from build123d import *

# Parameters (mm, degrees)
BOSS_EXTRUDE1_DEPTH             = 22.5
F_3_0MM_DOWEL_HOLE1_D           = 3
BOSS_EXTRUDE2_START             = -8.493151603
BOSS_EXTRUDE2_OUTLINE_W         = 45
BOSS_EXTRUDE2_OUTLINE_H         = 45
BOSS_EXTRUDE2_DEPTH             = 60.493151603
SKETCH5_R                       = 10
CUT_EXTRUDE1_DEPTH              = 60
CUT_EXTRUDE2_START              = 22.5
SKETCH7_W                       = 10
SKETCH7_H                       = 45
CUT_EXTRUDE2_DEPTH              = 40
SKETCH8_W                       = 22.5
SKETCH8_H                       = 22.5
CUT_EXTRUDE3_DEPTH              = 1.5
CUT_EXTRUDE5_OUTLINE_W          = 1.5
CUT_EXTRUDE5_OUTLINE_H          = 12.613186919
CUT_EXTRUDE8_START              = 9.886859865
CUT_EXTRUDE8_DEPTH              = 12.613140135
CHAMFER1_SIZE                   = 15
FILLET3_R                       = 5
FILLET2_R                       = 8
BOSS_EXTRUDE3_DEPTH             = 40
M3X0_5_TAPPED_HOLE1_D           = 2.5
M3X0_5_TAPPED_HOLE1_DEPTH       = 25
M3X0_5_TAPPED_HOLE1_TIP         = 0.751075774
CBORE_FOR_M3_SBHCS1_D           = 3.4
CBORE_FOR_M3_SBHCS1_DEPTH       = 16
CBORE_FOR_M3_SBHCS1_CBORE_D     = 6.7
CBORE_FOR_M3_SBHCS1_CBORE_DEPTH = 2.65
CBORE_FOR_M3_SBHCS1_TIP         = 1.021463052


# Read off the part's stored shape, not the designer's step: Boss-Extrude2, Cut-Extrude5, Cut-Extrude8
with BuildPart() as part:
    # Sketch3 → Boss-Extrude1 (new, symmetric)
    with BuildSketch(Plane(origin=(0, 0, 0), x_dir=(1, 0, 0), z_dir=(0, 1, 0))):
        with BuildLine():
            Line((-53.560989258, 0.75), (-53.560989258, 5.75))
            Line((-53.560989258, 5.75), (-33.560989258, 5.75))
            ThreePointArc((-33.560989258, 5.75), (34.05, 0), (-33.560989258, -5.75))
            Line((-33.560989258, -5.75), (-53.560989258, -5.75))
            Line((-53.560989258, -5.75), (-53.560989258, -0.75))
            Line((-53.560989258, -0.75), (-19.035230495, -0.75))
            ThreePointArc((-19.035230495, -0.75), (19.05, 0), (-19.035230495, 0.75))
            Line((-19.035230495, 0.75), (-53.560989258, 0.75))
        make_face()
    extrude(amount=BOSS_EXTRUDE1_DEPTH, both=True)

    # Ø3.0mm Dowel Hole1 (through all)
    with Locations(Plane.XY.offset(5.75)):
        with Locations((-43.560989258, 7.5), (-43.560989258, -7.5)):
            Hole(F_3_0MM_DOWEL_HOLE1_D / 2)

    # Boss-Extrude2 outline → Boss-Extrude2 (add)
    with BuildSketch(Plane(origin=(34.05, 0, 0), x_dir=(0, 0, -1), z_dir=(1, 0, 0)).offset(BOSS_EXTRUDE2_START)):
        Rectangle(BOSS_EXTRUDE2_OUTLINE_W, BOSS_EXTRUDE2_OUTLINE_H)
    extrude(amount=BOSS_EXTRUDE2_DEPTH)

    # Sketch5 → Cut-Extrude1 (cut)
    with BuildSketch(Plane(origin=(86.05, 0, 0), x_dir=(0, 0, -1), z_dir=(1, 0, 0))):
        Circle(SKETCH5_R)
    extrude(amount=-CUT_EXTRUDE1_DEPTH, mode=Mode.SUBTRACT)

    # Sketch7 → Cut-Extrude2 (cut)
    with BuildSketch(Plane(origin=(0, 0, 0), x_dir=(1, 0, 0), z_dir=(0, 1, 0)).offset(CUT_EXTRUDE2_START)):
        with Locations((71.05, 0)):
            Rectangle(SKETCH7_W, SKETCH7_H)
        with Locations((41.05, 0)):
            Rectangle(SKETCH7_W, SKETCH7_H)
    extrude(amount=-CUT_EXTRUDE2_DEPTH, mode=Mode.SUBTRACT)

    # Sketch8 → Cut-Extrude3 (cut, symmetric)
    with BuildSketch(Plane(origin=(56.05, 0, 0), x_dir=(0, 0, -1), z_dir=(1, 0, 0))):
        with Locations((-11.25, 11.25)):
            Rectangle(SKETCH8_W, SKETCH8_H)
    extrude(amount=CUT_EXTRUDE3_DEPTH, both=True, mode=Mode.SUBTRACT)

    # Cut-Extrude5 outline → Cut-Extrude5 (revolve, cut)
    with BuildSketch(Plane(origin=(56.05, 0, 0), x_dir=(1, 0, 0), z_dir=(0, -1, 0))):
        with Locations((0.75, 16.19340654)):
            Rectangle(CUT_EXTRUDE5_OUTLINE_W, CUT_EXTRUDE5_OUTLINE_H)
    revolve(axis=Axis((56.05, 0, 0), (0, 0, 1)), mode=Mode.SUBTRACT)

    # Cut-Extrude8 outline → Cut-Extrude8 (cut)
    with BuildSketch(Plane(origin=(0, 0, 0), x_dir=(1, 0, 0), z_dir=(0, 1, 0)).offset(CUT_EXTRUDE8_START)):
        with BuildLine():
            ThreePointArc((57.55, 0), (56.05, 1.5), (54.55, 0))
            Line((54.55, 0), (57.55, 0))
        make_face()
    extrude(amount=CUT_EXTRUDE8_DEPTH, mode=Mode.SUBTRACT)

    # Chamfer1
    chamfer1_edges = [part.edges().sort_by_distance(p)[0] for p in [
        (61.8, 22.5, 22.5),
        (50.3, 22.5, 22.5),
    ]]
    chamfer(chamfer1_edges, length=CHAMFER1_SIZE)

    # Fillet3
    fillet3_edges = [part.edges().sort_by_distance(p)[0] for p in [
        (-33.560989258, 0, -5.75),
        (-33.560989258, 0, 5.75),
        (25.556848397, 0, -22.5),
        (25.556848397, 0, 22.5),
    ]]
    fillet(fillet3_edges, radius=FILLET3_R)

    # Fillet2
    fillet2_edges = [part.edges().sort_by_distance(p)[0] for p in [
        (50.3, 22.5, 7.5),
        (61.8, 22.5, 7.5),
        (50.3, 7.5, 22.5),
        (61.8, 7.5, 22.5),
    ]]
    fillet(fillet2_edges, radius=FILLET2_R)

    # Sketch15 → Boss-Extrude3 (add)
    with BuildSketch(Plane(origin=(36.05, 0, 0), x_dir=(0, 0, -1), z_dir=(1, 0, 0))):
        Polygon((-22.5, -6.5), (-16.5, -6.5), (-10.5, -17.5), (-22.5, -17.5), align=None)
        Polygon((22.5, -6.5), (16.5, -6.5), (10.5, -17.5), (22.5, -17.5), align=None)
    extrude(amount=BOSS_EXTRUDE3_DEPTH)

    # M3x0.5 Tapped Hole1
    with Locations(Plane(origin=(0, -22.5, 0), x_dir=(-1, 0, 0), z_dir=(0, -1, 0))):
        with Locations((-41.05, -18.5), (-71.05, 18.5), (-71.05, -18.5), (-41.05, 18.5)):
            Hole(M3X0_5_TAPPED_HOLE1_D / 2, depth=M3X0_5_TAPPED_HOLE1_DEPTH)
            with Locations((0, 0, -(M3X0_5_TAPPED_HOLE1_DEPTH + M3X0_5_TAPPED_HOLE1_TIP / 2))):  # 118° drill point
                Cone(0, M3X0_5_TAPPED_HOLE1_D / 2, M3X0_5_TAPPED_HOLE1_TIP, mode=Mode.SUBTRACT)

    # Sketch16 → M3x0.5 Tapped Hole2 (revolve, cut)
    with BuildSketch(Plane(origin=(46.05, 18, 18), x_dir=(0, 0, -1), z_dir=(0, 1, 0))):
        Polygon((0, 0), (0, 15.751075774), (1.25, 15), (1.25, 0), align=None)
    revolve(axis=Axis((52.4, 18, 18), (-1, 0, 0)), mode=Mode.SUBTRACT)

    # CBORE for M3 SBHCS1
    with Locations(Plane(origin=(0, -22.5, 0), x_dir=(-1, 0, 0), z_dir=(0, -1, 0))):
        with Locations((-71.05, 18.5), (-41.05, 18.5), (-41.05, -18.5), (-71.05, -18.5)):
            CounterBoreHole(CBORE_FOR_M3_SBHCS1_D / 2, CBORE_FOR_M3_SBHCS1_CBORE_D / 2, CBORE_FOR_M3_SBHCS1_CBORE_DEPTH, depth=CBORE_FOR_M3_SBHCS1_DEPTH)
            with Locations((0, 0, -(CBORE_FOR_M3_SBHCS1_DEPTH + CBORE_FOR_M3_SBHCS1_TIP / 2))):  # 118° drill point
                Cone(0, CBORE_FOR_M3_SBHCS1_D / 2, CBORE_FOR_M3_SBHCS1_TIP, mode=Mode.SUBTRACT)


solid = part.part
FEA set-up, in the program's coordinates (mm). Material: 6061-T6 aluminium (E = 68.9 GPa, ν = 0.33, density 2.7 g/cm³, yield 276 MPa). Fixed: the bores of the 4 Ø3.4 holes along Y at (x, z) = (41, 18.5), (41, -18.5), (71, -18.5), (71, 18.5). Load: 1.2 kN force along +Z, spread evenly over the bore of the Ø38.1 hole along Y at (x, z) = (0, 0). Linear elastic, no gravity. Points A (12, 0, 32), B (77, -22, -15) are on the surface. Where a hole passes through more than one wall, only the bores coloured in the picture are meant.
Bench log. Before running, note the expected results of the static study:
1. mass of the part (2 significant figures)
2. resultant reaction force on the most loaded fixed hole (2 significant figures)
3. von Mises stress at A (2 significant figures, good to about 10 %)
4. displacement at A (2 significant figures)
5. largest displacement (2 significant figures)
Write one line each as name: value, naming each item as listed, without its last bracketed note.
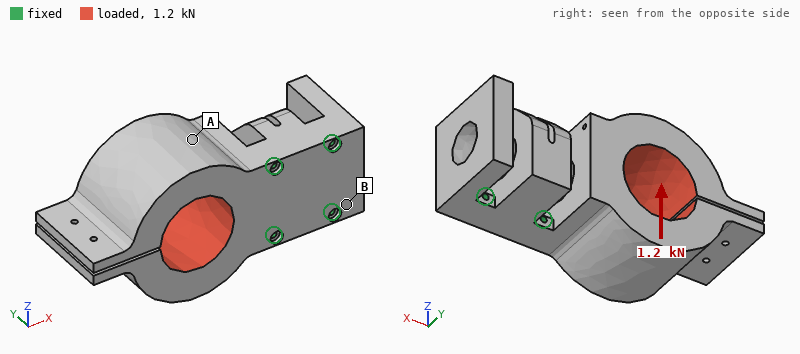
mass of the part: 490 g
resultant reaction force on the most loaded fixed hole: 1.4 kN
von Mises stress at A: 3.0 MPa
displacement at A: 11 µm
largest displacement: 40 µm
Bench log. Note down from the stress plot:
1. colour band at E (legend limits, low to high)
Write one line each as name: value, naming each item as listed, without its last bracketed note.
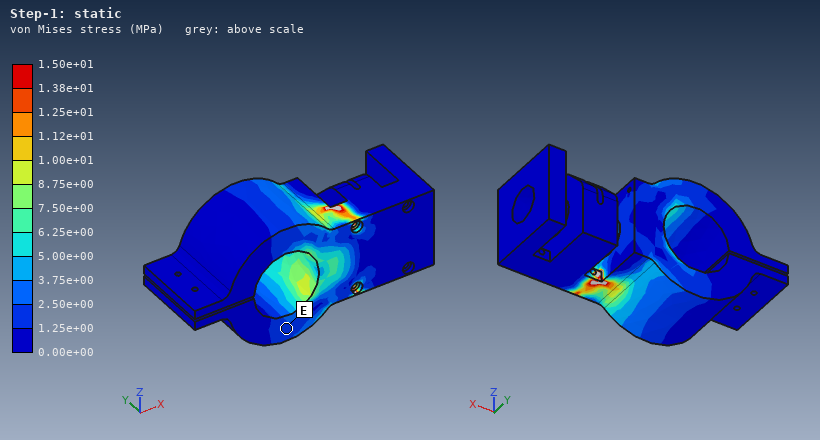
colour band at E: 1.25e+00 to 2.50e+00 MPa
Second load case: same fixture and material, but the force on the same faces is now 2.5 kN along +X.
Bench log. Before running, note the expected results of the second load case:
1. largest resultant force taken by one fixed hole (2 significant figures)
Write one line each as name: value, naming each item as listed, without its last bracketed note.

largest resultant force taken by one fixed hole: 1.5 kN
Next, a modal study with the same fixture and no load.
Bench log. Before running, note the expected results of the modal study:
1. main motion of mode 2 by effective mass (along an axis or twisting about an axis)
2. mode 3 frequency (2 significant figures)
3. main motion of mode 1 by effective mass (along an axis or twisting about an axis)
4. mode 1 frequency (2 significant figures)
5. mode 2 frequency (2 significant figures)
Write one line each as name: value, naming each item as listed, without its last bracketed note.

main motion of mode 2 by effective mass: along Z
mode 3 frequency: 2000 Hz
main motion of mode 1 by effective mass: along Y
mode 1 frequency: 1000 Hz
mode 2 frequency: 1700 Hz
